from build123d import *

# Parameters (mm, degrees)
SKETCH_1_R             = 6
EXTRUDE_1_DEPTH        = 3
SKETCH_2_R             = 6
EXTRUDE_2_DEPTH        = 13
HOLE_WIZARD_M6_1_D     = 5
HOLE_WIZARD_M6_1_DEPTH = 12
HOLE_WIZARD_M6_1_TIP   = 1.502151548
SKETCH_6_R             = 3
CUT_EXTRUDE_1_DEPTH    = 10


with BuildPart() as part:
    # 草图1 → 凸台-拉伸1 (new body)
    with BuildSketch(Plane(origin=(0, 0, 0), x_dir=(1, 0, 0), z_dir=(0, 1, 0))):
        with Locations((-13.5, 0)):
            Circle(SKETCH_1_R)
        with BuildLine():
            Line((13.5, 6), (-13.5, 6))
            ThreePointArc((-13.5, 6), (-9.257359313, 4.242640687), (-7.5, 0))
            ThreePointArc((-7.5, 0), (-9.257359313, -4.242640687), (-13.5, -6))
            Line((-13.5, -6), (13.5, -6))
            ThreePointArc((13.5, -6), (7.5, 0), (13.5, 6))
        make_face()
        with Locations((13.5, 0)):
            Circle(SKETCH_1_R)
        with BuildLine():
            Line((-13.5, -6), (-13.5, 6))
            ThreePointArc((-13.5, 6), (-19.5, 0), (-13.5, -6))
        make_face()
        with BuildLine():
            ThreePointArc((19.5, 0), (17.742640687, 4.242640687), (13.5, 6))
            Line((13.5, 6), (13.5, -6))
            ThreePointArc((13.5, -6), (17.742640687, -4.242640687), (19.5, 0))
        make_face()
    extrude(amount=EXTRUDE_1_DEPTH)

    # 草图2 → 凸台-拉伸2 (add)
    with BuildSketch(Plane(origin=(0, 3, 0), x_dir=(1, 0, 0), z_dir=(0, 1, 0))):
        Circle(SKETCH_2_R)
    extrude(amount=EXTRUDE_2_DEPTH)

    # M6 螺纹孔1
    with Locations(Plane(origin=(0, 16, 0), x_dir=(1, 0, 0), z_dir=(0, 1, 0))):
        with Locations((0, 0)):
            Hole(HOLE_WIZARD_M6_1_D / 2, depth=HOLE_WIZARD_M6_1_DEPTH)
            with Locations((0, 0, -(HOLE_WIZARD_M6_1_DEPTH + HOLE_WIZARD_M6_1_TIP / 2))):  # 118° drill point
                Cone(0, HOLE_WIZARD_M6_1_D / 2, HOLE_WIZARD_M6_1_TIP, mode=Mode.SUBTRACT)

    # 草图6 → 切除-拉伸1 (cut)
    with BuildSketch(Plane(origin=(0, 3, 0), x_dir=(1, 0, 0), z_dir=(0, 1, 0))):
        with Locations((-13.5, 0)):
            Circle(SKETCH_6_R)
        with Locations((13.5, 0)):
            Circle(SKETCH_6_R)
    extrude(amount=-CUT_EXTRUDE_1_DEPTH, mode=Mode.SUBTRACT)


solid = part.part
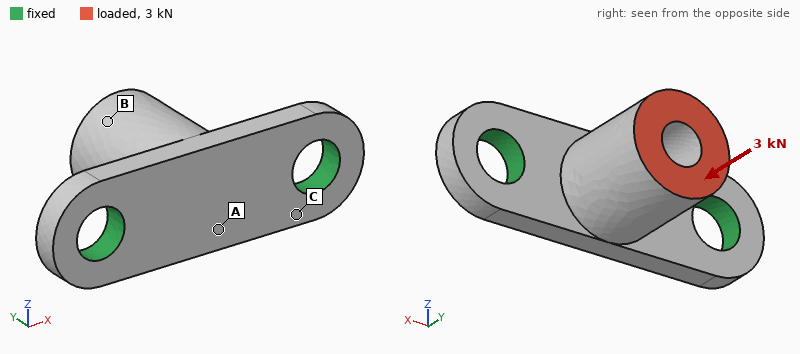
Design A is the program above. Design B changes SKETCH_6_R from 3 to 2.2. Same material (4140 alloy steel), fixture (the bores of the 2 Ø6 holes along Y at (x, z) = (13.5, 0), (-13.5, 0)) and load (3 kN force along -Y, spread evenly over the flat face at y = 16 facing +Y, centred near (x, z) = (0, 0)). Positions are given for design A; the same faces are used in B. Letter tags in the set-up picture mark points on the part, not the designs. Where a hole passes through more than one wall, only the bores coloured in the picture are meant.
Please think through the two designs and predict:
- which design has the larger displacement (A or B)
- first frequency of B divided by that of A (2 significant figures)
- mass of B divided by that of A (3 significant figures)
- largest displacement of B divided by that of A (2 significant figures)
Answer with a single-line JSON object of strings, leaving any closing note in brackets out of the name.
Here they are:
{"which design has the larger displacement": "B", "first frequency of B divided by that of A": "0.90", "mass of B divided by that of A": "1.03", "largest displacement of B divided by that of A": "1.3"}
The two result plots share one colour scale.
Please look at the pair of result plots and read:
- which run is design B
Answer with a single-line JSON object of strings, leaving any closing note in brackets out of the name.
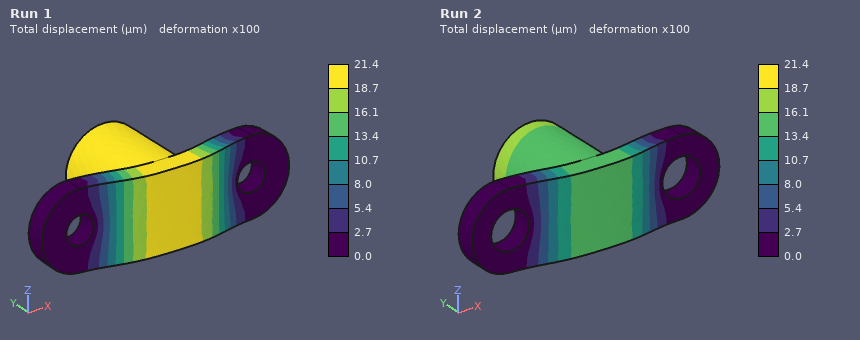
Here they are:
{"which run is design B": "Run 1"}
